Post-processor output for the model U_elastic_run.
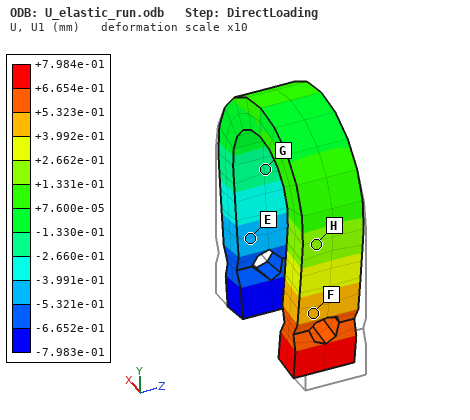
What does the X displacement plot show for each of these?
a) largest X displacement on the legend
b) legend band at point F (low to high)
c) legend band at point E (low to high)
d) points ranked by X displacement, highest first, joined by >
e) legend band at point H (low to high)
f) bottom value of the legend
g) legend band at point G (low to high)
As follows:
+7.984e-01 mm
+3.992e-01 to +5.323e-01 mm
-5.321e-01 to -3.991e-01 mm
F > H > G > E
+1.331e-01 to +2.662e-01 mm
-7.983e-01 mm
-2.660e-01 to -1.330e-01 mm
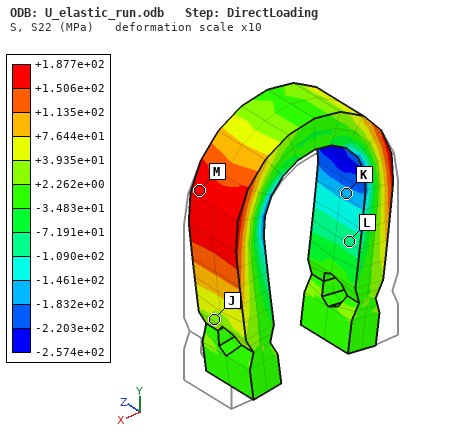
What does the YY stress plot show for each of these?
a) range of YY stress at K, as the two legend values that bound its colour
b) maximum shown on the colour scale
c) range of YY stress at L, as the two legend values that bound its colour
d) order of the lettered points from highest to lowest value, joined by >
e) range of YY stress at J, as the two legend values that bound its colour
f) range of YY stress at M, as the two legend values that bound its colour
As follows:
-1.832e+02 to -1.461e+02 MPa
+1.877e+02 MPa
-1.090e+02 to -7.191e+01 MPa
M > J > L > K
+2.262e+00 to +3.935e+01 MPa
+1.506e+02 to +1.877e+02 MPa
